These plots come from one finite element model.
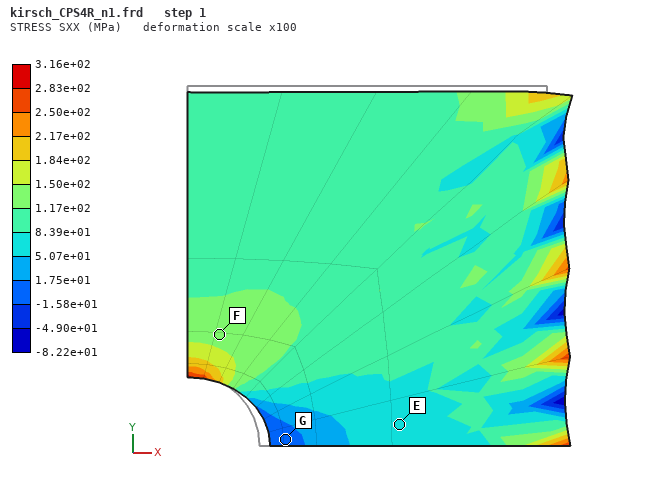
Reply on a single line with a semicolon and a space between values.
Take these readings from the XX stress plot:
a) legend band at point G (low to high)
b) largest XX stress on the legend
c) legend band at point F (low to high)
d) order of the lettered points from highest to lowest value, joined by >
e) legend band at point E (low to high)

-1.58e+01 to 1.75e+01 MPa; 3.16e+02 MPa; 1.17e+02 to 1.50e+02 MPa; F > E > G; 5.07e+01 to 8.39e+01 MPa
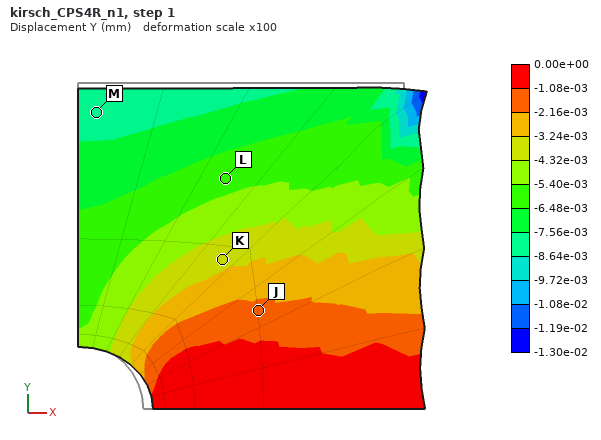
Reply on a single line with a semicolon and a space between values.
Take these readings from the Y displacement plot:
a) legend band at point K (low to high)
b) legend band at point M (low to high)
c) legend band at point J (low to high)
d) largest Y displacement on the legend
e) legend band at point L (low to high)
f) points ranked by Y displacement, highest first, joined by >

-4.32e-03 to -3.24e-03 mm; -8.64e-03 to -7.56e-03 mm; -2.16e-03 to -1.08e-03 mm; 0.00e+00 mm; -6.48e-03 to -5.40e-03 mm; J > K > L > M
